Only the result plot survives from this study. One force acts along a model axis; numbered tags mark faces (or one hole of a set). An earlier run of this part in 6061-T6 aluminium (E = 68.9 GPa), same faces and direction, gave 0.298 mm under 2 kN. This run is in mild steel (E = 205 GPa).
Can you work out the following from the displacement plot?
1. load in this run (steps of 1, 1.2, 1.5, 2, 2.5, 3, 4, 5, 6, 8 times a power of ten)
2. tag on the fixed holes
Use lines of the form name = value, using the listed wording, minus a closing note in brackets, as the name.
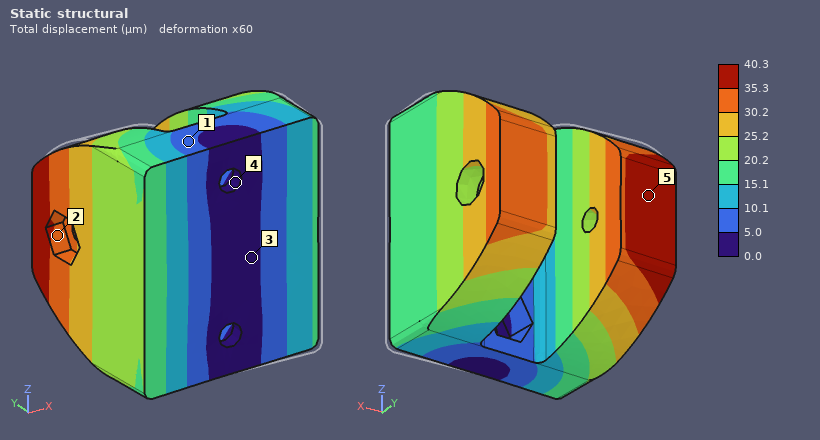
load in this run = 800 N
tag on the fixed holes = 4
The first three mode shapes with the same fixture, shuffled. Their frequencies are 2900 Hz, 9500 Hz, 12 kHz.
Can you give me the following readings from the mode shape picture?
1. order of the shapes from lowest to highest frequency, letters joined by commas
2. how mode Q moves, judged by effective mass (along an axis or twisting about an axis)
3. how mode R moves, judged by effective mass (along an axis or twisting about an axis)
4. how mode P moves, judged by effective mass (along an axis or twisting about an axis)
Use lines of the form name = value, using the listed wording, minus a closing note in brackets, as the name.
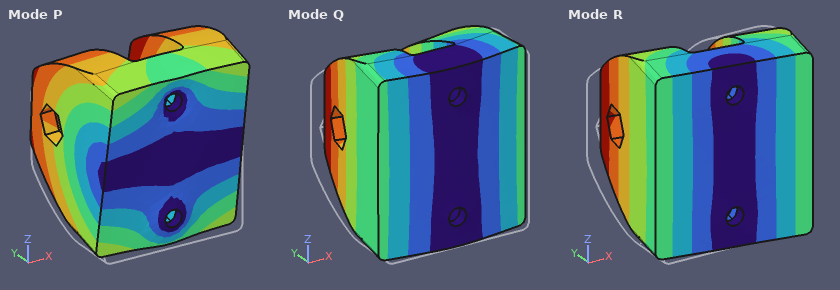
order of the shapes from lowest to highest frequency, letters joined by commas = R, Q, P
how mode Q moves, judged by effective mass = along Y
how mode R moves, judged by effective mass = along X
how mode P moves, judged by effective mass = along Z
